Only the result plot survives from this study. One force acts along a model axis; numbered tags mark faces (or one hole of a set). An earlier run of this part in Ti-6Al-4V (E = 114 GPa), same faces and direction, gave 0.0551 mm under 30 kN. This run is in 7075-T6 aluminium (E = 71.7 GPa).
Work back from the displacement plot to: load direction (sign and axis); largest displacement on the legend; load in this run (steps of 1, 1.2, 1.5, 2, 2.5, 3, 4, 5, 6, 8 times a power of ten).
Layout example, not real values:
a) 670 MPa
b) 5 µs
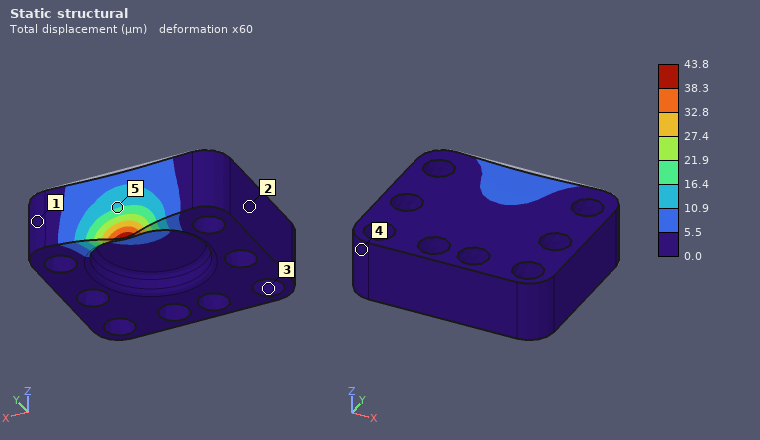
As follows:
a) -Y
b) 43.8 µm
c) 15 kN
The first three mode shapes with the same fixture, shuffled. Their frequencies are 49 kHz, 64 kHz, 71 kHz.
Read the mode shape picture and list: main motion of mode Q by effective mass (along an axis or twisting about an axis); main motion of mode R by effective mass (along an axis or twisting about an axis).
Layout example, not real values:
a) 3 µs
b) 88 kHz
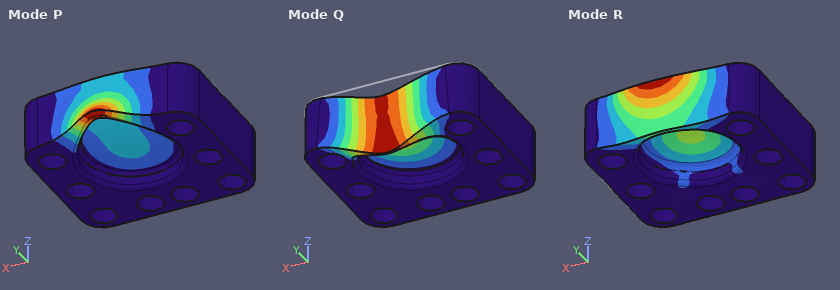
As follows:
a) along Z
b) along Y
